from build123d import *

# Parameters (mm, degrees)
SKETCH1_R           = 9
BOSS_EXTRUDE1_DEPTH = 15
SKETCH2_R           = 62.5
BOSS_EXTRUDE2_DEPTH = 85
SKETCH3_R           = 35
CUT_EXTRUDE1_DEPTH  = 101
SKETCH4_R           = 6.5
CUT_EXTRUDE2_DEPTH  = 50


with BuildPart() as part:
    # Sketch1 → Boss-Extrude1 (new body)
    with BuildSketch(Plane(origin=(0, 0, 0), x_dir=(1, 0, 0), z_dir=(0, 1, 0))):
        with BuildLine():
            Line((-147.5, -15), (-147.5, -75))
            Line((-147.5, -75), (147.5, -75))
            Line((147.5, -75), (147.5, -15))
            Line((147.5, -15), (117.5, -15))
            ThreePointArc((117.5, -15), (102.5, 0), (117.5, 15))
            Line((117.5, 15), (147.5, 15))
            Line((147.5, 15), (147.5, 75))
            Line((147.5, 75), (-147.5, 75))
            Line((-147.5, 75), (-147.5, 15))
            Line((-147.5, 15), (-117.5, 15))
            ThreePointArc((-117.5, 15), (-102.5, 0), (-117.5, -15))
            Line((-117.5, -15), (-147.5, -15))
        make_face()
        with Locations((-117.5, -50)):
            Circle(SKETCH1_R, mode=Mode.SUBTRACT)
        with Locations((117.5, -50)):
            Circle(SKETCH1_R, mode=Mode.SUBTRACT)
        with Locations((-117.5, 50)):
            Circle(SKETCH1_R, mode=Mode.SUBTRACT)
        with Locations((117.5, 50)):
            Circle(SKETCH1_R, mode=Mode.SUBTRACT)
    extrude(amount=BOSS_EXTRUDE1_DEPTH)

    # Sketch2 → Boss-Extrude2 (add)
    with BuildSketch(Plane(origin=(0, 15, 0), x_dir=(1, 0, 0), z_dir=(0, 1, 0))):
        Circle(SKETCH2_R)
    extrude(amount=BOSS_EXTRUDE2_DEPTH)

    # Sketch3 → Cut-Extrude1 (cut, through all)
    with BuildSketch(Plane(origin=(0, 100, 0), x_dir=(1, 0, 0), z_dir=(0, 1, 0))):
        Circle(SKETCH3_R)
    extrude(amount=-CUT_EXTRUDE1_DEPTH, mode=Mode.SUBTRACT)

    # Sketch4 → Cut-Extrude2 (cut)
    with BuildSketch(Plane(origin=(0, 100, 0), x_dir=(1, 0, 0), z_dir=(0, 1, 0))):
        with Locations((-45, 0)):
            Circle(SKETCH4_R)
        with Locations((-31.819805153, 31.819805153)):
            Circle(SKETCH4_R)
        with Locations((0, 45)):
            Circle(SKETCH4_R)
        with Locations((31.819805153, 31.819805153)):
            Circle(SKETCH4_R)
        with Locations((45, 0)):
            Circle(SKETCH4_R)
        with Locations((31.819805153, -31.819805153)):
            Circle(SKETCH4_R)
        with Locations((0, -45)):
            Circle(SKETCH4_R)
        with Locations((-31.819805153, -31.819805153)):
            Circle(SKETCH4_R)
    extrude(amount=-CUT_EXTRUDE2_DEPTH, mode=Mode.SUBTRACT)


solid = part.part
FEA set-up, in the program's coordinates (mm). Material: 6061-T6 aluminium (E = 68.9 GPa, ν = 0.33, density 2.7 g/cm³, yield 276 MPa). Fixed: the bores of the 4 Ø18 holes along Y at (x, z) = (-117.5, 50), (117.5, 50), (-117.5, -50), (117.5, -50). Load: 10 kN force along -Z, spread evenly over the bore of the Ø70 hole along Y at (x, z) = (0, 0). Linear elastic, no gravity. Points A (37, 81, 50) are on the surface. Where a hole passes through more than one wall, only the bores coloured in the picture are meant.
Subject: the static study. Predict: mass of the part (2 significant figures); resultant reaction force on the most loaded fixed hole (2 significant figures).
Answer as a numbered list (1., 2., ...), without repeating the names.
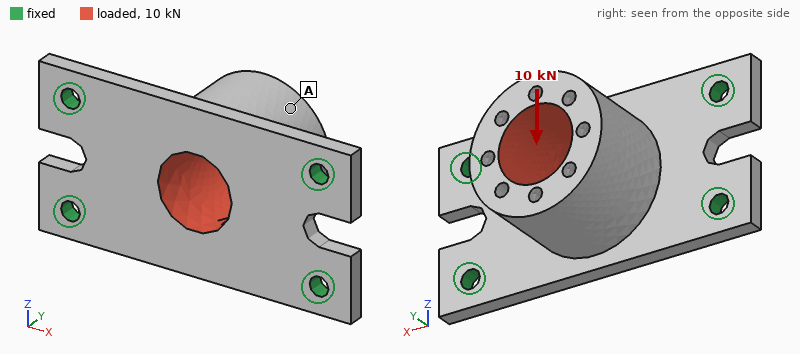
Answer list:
1. 3.3 kg
2. 4.1 kN
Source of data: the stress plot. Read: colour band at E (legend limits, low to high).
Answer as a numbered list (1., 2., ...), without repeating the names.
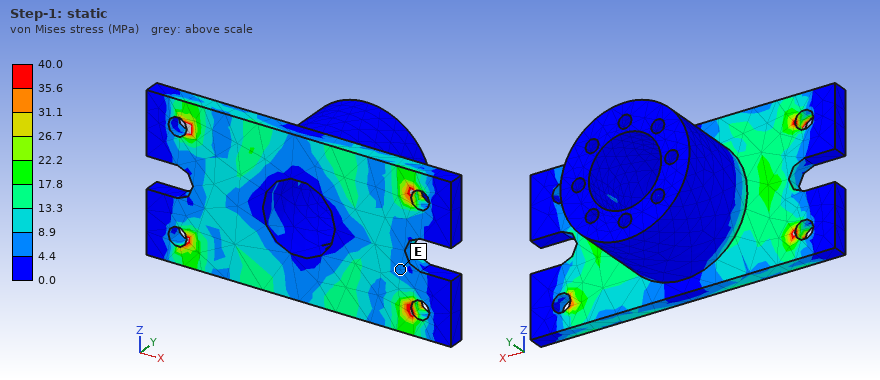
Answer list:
1. 4.4 to 8.9 MPa
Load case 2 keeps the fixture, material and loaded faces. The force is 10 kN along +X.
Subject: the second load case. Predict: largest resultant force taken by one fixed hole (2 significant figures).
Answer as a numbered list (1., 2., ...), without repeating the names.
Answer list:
1. 2.9 kN
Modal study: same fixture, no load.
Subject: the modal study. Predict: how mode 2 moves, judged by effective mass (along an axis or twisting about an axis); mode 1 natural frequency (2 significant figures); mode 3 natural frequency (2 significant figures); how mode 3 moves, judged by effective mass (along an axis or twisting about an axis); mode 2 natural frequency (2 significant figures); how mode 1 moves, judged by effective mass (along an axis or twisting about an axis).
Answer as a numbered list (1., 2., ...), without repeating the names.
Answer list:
1. along Y
2. 980 Hz
3. 1800 Hz
4. along X
5. 1200 Hz
6. along Z
